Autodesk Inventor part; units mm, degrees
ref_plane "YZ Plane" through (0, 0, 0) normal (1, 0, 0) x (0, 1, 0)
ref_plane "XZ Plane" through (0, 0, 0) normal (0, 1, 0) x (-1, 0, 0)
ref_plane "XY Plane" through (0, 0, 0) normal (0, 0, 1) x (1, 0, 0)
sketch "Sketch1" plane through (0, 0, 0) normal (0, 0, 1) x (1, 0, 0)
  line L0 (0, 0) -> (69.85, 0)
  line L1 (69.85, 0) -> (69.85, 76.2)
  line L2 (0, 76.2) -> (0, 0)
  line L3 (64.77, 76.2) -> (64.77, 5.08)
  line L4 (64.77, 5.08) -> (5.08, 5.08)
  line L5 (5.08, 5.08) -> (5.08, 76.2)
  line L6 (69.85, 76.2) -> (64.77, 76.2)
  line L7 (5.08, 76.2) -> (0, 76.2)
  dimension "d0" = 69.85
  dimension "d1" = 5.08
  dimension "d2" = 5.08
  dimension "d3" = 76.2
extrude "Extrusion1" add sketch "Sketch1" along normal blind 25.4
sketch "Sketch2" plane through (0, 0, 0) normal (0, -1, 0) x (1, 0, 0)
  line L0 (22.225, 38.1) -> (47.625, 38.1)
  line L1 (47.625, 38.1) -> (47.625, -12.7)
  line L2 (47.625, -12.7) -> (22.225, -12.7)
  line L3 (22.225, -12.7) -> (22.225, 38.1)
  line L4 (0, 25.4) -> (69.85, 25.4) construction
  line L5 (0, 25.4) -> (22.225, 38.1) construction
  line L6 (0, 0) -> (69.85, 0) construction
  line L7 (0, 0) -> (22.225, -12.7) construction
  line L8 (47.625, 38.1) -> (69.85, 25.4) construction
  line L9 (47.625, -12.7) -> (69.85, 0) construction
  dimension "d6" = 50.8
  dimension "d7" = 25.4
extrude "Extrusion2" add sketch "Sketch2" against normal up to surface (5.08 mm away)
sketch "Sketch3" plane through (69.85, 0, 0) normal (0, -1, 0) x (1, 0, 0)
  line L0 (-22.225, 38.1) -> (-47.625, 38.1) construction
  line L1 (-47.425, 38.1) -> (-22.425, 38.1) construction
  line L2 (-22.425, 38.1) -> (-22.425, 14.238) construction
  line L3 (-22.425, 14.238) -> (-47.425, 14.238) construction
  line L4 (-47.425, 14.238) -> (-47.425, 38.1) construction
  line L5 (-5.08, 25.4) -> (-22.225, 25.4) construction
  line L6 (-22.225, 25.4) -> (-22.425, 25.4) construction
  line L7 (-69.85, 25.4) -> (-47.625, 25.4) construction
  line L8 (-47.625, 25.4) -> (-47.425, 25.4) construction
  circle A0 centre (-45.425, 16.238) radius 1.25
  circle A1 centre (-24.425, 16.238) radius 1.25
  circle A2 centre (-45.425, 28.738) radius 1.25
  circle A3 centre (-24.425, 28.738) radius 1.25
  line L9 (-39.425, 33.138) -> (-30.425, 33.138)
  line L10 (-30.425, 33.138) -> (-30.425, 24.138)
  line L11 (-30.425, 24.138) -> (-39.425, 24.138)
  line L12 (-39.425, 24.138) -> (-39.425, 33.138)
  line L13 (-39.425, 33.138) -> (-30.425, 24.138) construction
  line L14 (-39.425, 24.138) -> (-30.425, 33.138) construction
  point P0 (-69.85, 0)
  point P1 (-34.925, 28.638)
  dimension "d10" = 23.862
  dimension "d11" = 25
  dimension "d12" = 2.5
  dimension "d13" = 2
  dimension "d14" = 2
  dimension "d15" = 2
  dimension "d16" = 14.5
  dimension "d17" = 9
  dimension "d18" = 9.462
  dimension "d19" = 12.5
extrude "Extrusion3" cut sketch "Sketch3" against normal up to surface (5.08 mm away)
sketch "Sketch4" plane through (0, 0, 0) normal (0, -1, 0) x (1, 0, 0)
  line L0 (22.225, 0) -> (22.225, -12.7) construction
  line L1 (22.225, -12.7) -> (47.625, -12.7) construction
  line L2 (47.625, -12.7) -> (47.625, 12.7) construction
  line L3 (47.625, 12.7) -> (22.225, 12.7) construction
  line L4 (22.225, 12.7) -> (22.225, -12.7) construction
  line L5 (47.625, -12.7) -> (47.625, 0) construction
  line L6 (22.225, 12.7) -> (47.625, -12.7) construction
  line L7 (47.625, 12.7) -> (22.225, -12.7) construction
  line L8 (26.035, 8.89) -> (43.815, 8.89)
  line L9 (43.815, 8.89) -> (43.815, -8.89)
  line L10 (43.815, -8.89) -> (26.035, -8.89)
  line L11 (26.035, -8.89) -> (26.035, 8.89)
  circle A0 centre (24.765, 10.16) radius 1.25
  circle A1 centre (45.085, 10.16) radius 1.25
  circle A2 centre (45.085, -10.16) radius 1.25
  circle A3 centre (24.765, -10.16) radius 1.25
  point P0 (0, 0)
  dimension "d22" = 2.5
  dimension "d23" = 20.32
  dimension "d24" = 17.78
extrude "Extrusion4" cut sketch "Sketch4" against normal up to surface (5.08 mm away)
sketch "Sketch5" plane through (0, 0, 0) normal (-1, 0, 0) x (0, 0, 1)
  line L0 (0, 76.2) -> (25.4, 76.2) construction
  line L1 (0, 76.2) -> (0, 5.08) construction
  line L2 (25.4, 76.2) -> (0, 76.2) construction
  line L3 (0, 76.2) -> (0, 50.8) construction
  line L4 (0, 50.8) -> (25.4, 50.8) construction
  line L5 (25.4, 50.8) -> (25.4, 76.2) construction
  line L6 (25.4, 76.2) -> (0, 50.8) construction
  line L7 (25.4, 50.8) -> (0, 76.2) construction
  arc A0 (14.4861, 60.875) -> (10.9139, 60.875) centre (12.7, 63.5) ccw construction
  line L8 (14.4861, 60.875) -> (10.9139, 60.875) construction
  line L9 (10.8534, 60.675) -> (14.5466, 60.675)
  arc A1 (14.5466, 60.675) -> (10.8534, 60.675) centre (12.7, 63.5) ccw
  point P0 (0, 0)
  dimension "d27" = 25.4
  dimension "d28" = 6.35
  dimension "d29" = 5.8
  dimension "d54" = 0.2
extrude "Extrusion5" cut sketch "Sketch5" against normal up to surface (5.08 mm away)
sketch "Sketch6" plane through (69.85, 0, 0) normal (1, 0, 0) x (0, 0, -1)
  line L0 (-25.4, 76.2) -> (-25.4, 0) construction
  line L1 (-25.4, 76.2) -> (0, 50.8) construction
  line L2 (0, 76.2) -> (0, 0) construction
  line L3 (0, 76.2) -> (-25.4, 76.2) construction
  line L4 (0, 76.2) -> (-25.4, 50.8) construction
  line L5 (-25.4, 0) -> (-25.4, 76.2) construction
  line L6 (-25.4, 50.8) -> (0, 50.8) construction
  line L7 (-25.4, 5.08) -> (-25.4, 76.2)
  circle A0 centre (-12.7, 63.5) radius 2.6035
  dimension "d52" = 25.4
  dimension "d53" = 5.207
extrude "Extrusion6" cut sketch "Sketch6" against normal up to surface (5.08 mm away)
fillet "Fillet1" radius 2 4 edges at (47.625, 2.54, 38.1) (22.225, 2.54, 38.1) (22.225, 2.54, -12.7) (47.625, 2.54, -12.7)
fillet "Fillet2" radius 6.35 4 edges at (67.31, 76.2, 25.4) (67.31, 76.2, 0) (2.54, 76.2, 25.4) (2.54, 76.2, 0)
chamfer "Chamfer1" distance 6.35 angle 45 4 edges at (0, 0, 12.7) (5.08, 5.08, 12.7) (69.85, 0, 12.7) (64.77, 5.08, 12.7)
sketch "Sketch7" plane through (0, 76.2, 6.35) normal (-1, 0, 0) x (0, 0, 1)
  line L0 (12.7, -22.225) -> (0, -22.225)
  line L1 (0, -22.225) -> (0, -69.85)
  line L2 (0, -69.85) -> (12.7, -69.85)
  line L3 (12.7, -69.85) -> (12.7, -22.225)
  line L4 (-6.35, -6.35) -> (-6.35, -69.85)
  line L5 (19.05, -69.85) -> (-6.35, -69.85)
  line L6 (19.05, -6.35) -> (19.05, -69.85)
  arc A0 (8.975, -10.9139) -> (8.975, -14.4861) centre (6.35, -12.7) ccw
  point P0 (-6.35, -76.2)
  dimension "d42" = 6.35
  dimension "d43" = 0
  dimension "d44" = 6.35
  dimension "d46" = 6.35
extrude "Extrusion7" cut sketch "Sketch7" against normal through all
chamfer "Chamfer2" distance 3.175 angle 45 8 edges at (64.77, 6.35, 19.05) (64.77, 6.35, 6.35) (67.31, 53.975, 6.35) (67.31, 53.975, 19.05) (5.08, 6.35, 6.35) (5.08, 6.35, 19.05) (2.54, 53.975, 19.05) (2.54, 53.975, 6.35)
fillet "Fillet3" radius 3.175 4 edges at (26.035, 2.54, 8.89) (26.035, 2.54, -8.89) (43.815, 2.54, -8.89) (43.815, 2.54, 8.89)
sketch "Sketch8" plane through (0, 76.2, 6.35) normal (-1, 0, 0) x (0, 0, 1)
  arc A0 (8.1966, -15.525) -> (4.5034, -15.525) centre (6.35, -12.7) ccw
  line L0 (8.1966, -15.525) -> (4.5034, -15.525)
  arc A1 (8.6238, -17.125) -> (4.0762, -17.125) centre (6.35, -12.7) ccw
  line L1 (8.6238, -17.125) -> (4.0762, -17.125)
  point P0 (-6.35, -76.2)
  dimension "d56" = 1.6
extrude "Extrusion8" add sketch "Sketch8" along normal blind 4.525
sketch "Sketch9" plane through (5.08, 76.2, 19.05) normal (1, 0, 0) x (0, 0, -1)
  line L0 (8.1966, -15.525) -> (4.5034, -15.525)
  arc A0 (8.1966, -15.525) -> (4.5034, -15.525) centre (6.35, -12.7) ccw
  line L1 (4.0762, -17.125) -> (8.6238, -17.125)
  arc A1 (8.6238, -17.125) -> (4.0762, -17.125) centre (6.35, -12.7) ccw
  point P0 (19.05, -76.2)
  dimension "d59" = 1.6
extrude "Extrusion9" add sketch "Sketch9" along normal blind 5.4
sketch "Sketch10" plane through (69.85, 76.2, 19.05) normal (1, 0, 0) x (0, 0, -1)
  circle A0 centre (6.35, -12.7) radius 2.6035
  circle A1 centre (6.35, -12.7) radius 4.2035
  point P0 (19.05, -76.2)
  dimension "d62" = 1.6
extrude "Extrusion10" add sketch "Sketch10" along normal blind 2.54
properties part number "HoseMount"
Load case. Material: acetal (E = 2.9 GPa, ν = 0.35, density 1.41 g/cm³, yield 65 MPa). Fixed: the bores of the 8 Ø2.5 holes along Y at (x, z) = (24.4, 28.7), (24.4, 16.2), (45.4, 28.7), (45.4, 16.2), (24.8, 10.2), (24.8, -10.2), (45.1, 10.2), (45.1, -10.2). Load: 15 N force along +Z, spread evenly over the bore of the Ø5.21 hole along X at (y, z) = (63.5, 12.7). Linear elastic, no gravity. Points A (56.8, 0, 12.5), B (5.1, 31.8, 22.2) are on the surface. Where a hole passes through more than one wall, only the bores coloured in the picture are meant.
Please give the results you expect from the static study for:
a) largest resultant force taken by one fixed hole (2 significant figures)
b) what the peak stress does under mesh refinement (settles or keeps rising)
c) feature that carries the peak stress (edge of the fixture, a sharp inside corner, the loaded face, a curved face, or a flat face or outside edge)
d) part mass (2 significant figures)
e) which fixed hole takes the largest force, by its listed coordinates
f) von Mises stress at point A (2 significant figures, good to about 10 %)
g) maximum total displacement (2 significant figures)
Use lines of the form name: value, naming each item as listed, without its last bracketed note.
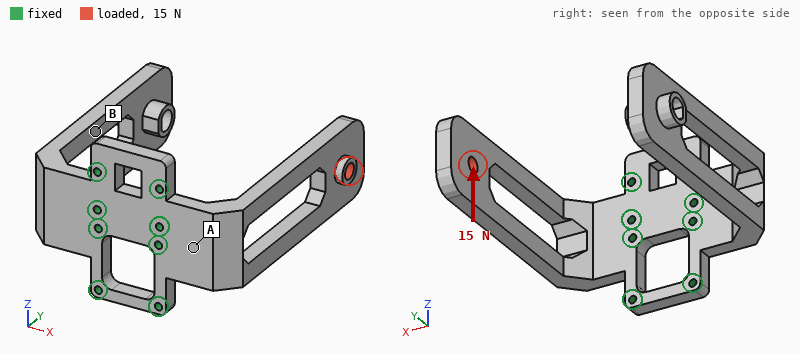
largest resultant force taken by one fixed hole: 43 N
what the peak stress does under mesh refinement: keeps rising
feature that carries the peak stress: edge of the fixture
part mass: 31 g
which fixed hole takes the largest force, by its listed coordinates: (45.1, 10.2)
von Mises stress at point A: 4.9 MPa
maximum total displacement: 1.1 mm
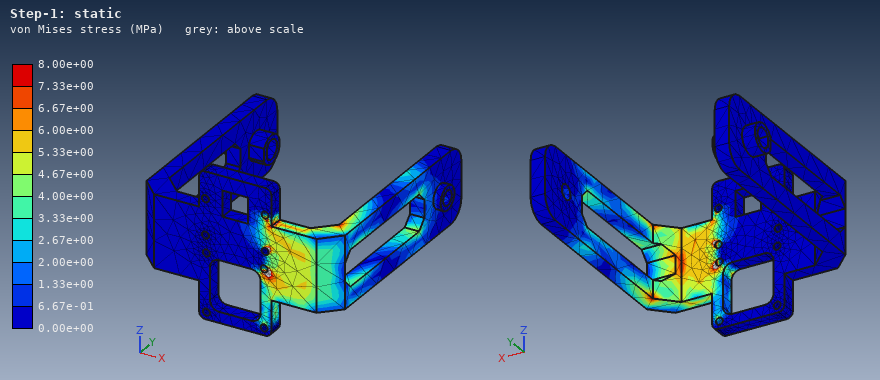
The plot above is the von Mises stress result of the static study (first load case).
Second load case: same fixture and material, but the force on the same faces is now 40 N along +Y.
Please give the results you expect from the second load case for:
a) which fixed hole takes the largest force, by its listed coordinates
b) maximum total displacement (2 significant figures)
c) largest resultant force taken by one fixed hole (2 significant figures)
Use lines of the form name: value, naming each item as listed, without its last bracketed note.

which fixed hole takes the largest force, by its listed coordinates: (45.4, 16.2)
maximum total displacement: 1.3 mm
largest resultant force taken by one fixed hole: 33 N
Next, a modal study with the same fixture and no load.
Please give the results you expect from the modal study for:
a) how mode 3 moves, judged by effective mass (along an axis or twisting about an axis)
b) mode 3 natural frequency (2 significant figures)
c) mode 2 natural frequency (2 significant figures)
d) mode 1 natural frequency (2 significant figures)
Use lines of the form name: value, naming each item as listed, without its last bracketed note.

how mode 3 moves, judged by effective mass: along Z
mode 3 natural frequency: 260 Hz
mode 2 natural frequency: 150 Hz
mode 1 natural frequency: 150 Hz
